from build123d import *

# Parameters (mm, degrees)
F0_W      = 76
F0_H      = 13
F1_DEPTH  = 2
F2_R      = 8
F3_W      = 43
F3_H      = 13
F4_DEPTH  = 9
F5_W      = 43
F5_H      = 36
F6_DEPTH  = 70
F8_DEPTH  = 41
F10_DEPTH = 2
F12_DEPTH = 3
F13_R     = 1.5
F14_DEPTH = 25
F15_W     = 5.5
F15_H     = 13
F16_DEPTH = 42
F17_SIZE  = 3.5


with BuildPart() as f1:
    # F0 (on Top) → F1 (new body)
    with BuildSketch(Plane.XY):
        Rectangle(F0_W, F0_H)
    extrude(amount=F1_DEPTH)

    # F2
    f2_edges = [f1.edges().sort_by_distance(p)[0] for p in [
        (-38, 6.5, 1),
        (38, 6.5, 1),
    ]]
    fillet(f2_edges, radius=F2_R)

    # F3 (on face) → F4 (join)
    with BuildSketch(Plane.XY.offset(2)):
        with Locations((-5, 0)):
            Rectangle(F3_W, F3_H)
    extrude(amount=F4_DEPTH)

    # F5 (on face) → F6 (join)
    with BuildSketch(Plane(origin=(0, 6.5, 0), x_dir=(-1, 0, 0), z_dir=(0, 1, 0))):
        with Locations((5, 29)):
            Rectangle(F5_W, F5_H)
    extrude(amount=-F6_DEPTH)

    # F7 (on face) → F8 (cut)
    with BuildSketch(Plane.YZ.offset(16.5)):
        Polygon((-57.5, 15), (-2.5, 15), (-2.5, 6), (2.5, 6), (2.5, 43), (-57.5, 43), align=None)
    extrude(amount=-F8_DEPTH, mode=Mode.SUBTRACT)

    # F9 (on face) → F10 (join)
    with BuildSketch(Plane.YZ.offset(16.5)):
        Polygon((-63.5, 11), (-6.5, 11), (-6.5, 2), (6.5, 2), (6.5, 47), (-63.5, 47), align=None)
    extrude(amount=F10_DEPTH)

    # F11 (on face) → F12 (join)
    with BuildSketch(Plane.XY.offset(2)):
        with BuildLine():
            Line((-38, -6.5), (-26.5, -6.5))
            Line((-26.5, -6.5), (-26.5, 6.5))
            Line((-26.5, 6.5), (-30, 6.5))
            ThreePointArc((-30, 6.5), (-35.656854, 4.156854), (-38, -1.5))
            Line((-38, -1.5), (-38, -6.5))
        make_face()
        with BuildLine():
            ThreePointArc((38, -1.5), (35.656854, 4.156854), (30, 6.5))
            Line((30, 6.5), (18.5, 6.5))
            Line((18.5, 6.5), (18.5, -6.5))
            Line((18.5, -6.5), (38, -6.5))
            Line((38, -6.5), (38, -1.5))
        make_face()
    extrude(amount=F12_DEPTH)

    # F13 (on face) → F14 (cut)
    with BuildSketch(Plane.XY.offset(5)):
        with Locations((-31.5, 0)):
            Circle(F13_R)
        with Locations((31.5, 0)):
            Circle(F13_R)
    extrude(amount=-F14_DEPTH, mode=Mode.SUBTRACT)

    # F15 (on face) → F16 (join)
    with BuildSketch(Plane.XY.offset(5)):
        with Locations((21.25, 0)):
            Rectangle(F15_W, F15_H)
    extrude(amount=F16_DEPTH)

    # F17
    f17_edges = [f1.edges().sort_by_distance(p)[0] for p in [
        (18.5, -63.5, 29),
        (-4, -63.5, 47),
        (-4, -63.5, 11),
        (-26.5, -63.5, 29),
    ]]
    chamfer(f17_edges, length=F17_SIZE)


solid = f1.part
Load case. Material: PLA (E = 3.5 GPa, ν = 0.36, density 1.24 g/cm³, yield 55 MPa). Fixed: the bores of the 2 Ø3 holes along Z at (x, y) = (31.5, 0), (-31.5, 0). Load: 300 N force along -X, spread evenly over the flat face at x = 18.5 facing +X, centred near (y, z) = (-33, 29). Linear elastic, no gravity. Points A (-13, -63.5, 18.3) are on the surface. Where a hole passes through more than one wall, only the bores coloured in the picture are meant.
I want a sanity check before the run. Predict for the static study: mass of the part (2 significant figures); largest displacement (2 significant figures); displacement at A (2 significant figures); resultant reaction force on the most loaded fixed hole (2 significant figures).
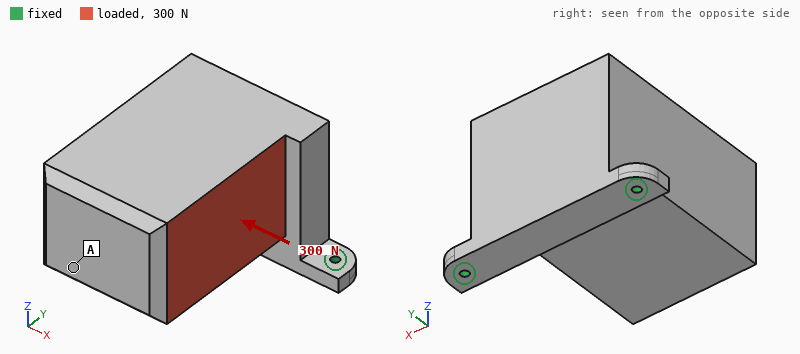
66 g
0.49 mm
0.42 mm
270 N
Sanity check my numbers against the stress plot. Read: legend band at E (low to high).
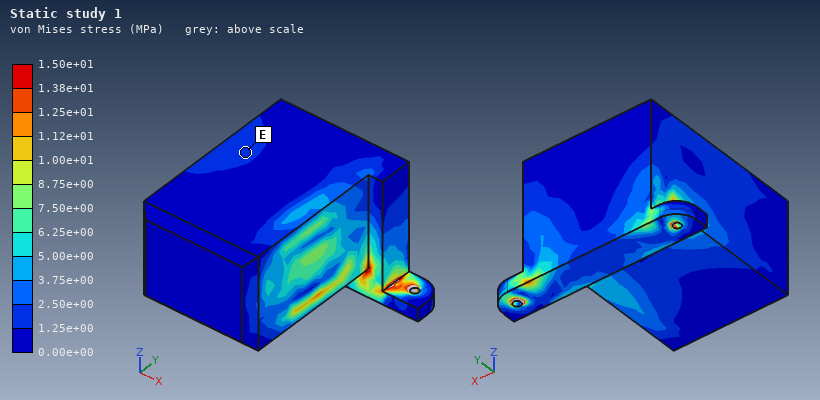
1.25e+00 to 2.50e+00 MPa
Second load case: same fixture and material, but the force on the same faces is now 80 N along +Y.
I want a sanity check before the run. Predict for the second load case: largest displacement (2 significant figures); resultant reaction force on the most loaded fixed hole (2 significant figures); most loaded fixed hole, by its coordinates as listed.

1.2 mm
66 N
(31.5, 0)
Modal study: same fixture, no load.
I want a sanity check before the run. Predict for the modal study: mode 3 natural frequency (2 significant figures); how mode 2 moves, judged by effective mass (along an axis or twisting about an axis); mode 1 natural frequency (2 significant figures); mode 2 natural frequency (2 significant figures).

1200 Hz
along X
160 Hz
640 Hz
